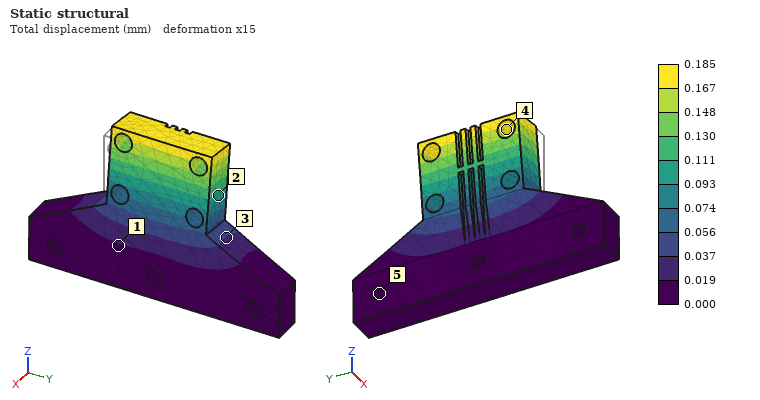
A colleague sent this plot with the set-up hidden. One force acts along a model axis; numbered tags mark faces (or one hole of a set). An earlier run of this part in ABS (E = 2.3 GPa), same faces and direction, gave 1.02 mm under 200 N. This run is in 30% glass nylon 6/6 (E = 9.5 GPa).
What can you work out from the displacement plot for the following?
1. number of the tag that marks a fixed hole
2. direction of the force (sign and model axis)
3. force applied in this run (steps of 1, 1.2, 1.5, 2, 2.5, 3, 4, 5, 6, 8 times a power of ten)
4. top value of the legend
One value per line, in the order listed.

5
-X
150 N
0.185 mm
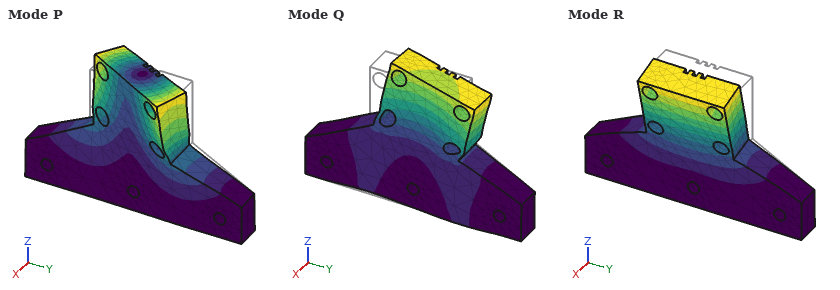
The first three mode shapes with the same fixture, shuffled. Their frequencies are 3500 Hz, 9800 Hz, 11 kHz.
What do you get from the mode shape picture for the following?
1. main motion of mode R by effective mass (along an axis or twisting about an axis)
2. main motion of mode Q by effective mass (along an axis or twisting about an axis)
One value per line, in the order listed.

along X
along Y
